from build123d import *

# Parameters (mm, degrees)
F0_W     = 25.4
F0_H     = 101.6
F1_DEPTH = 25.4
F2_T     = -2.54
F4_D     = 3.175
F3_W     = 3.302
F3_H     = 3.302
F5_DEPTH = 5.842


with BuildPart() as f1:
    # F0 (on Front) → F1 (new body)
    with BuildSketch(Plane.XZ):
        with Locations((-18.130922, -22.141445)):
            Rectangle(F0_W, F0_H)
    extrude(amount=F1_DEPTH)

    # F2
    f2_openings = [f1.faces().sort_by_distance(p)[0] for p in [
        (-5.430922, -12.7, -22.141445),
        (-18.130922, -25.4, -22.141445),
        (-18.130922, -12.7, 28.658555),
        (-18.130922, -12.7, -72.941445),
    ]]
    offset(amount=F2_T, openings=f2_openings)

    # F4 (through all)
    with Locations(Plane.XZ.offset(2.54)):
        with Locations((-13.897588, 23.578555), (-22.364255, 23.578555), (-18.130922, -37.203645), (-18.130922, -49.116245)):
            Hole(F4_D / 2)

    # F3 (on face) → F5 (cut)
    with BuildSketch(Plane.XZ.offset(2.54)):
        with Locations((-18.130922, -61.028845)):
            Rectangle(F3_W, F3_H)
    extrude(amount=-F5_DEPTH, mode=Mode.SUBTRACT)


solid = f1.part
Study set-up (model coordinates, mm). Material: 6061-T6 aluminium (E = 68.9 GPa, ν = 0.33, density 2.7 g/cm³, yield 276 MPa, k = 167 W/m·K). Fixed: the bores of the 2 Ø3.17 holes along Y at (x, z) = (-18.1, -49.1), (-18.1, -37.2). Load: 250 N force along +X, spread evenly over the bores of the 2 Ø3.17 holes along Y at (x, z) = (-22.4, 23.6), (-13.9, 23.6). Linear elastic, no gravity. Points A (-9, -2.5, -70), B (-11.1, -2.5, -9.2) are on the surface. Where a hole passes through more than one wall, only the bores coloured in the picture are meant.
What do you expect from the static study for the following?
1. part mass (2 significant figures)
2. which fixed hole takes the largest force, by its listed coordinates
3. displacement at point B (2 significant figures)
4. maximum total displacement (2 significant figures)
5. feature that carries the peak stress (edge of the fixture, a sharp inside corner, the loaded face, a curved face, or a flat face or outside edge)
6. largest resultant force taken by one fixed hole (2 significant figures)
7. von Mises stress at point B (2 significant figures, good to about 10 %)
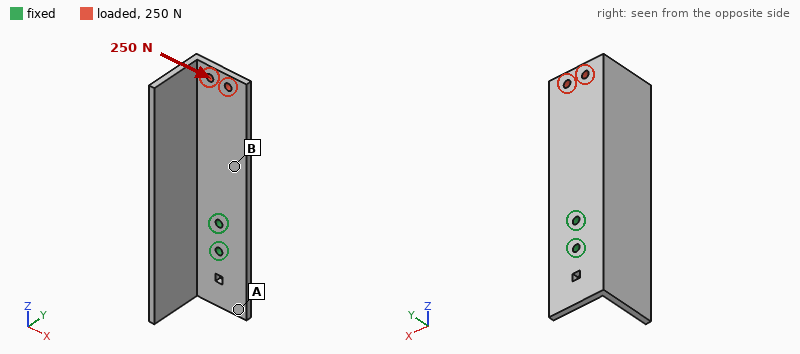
33 g
(-18.1, -37.2)
0.055 mm
0.16 mm
edge of the fixture
1.2 kN
17 MPa
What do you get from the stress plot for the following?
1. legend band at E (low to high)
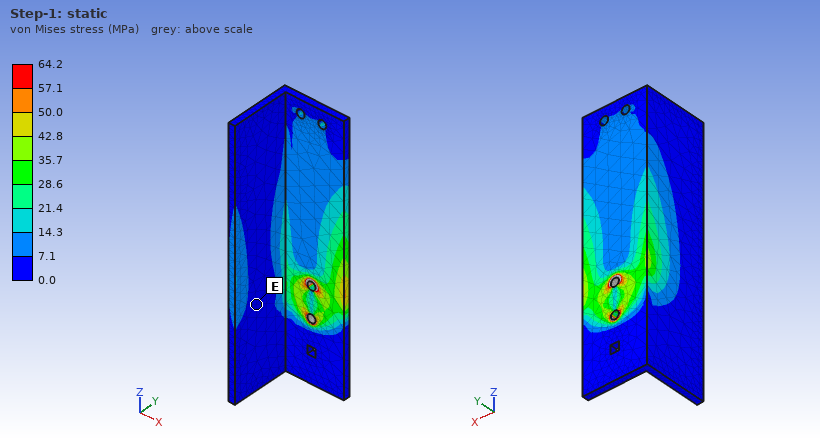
0.0 to 7.1 MPa
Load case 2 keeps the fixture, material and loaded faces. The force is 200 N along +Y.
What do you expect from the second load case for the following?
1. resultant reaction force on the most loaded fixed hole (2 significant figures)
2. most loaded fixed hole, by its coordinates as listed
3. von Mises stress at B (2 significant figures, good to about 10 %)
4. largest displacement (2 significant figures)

810 N
(-18.1, -37.2)
36 MPa
1.0 mm
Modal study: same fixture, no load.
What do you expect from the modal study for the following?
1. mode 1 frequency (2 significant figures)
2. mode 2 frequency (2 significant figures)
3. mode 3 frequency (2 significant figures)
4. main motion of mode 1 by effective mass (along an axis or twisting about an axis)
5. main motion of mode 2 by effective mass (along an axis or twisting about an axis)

870 Hz
1200 Hz
2200 Hz
along Y
along X
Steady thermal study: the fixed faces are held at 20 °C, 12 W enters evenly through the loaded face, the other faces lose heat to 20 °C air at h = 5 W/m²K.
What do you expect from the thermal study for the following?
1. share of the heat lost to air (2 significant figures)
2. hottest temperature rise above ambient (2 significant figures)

7.4 %
50 K
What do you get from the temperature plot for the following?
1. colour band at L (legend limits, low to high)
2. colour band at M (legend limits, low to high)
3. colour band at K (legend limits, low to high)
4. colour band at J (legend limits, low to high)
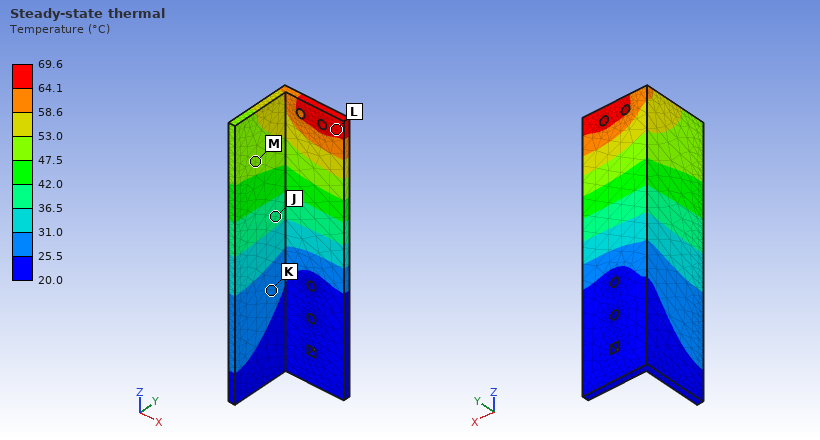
64.1 to 69.6 °C
47.5 to 53.0 °C
25.5 to 31.0 °C
36.5 to 42.0 °C
